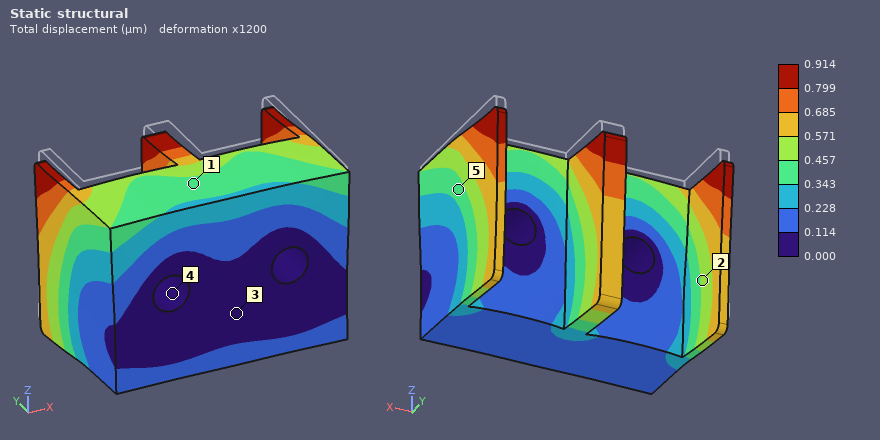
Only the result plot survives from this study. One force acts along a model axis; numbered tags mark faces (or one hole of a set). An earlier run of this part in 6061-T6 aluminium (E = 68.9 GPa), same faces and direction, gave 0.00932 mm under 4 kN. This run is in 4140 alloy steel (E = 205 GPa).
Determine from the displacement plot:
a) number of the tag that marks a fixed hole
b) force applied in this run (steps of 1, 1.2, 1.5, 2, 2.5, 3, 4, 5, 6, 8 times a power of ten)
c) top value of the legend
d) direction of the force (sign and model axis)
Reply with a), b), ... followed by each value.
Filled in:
a) 4
b) 1.2 kN
c) 0.914 µm
d) -Z
